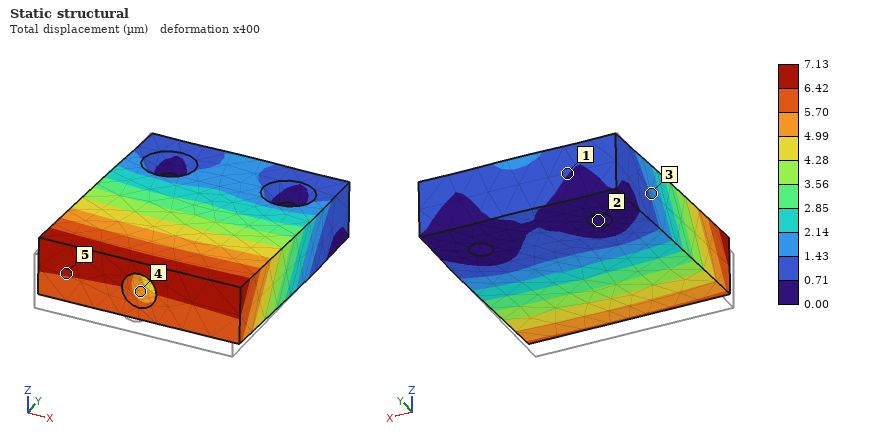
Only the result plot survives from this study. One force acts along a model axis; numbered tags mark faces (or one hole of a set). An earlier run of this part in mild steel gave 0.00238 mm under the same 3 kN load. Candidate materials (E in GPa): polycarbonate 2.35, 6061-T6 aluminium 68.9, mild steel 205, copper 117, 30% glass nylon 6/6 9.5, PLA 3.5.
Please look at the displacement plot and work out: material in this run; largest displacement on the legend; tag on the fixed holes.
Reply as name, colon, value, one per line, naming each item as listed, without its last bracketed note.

material in this run: 6061-T6 aluminium
largest displacement on the legend: 7.13 µm
tag on the fixed holes: 2
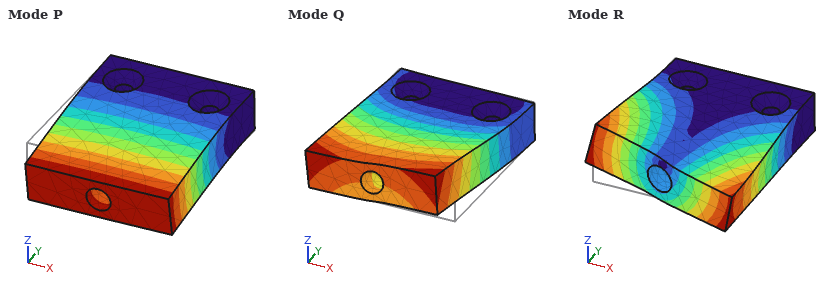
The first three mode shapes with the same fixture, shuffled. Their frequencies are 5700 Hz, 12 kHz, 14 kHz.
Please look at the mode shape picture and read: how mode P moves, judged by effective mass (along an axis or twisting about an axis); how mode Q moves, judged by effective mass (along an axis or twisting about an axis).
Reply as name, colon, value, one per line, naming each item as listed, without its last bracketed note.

how mode P moves, judged by effective mass: along Z
how mode Q moves, judged by effective mass: along X
